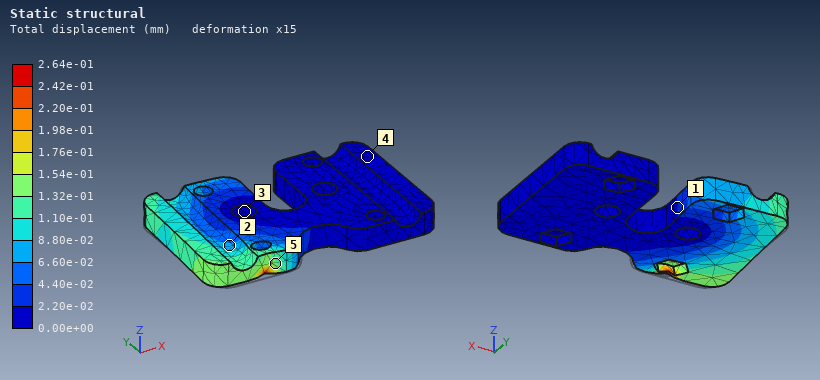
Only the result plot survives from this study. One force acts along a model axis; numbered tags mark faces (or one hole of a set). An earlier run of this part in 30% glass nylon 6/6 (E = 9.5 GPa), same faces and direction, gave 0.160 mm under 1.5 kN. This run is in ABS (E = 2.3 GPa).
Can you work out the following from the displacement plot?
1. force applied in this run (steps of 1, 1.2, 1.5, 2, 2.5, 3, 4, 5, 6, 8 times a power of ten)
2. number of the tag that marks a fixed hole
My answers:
600 N
3
